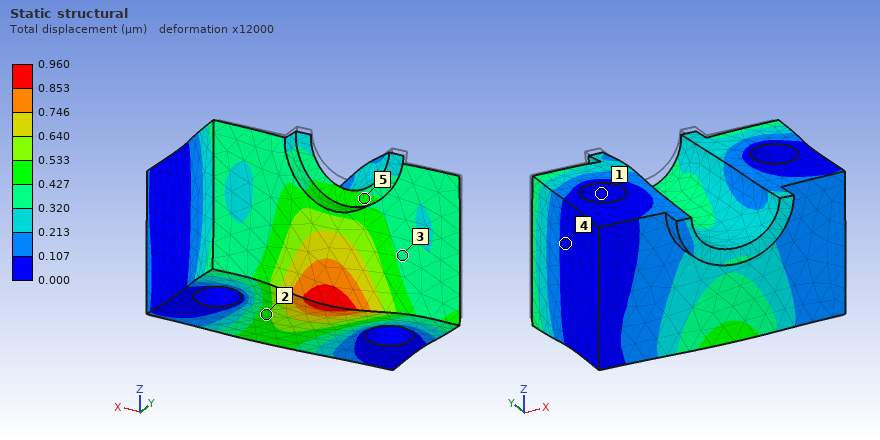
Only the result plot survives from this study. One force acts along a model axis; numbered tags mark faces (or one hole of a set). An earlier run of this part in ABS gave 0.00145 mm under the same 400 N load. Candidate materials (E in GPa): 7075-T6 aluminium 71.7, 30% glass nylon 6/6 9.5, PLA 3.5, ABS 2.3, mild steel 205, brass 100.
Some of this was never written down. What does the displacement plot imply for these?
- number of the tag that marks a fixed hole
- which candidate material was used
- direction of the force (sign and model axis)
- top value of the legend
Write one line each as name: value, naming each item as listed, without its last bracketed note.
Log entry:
number of the tag that marks a fixed hole: 1
which candidate material was used: PLA
direction of the force: -Y
top value of the legend: 0.960 µm
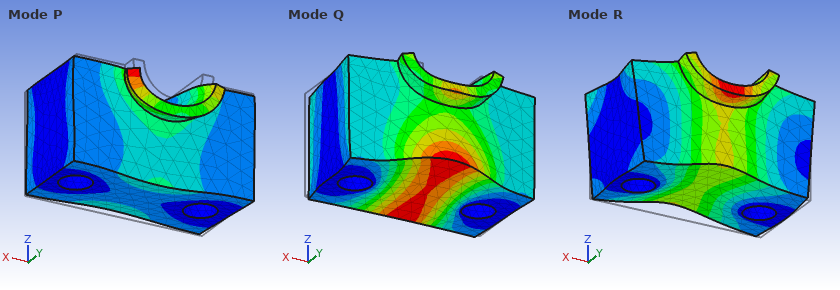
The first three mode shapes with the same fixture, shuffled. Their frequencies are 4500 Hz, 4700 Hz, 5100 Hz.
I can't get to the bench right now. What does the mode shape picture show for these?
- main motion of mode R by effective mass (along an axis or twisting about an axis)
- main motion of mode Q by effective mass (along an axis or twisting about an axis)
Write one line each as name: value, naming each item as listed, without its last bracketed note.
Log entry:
main motion of mode R by effective mass: along Z
main motion of mode Q by effective mass: along Y
